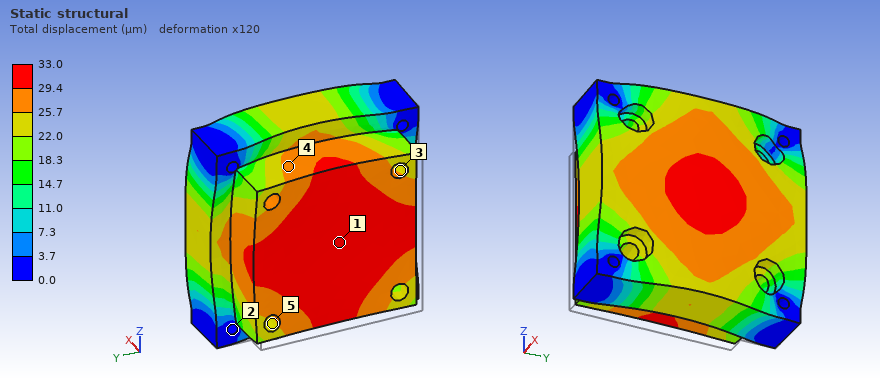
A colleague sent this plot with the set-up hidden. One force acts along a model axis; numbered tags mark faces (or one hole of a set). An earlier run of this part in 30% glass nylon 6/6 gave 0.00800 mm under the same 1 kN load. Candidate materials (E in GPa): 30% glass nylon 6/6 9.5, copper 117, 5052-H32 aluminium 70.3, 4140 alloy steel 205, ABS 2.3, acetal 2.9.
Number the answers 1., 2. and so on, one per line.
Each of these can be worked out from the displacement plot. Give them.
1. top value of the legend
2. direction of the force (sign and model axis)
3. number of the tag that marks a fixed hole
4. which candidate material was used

1. 33.0 µm
2. +X
3. 2
4. ABS
